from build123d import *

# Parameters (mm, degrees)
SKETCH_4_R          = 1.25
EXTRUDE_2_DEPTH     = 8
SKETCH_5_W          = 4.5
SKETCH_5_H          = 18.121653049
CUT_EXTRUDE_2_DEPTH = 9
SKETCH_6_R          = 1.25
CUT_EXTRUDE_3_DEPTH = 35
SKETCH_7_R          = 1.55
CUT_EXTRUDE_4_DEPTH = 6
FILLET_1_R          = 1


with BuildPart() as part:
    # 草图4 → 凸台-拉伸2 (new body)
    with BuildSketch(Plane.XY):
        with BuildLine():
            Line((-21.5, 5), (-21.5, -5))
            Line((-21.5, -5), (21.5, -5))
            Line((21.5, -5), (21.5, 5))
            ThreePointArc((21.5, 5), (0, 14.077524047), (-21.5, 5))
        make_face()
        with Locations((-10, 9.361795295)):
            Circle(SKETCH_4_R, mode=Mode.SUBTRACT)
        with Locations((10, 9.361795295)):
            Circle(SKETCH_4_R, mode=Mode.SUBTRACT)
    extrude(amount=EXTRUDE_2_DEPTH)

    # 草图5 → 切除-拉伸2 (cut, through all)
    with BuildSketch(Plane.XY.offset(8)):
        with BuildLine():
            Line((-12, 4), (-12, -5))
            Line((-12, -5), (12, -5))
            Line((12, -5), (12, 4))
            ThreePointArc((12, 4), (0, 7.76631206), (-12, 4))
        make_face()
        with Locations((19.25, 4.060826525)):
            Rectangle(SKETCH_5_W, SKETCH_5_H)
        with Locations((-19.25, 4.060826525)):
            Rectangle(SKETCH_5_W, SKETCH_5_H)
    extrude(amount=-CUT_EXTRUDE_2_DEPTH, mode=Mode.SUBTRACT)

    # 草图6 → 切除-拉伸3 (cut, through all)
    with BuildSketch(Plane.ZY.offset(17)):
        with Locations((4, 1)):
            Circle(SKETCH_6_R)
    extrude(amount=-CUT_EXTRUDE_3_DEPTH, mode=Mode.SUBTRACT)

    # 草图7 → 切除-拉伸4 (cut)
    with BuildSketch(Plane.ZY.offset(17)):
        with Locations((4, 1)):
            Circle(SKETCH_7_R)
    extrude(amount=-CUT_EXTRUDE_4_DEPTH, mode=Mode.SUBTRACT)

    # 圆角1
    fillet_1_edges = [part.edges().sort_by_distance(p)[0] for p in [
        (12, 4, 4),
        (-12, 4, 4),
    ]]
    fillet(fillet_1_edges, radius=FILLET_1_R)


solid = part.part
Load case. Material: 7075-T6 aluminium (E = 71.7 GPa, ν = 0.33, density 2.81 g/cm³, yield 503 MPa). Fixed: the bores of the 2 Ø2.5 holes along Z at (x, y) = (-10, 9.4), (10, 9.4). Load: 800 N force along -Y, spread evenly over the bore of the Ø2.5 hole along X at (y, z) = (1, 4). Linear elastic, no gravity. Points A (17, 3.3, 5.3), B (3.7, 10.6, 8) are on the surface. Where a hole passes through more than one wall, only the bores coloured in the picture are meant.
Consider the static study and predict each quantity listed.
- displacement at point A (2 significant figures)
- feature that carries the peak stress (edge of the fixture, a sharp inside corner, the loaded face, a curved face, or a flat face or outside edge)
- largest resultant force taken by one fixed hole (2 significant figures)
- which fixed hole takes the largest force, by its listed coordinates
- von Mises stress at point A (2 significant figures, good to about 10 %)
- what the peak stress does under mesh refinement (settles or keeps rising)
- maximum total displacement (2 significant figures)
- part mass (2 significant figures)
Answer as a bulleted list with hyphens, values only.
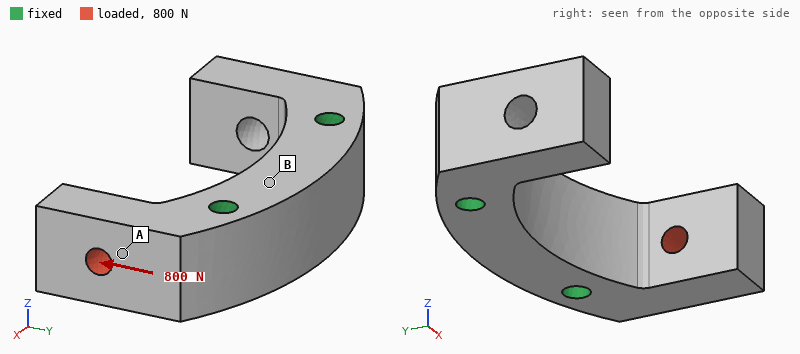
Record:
- 13 µm
- edge of the fixture
- 850 N
- (10, 9.4)
- 27 MPa
- keeps rising
- 22 µm
- 6.7 g
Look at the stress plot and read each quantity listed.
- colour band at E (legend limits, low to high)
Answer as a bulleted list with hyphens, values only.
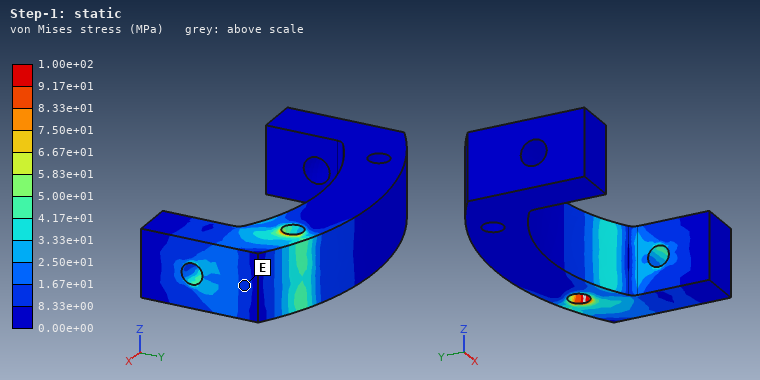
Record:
- 8.33e+00 to 1.67e+01 MPa
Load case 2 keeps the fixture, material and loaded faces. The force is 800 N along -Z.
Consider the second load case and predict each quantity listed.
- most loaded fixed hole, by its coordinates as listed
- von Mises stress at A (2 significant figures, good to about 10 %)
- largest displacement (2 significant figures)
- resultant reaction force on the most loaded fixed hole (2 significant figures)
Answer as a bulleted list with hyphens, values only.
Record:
- (10, 9.4)
- 29 MPa
- 38 µm
- 820 N
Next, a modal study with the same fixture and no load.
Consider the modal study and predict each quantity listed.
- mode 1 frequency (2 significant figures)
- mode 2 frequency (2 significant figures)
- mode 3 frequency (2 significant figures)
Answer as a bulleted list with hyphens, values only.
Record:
- 18 kHz
- 19 kHz
- 23 kHz
